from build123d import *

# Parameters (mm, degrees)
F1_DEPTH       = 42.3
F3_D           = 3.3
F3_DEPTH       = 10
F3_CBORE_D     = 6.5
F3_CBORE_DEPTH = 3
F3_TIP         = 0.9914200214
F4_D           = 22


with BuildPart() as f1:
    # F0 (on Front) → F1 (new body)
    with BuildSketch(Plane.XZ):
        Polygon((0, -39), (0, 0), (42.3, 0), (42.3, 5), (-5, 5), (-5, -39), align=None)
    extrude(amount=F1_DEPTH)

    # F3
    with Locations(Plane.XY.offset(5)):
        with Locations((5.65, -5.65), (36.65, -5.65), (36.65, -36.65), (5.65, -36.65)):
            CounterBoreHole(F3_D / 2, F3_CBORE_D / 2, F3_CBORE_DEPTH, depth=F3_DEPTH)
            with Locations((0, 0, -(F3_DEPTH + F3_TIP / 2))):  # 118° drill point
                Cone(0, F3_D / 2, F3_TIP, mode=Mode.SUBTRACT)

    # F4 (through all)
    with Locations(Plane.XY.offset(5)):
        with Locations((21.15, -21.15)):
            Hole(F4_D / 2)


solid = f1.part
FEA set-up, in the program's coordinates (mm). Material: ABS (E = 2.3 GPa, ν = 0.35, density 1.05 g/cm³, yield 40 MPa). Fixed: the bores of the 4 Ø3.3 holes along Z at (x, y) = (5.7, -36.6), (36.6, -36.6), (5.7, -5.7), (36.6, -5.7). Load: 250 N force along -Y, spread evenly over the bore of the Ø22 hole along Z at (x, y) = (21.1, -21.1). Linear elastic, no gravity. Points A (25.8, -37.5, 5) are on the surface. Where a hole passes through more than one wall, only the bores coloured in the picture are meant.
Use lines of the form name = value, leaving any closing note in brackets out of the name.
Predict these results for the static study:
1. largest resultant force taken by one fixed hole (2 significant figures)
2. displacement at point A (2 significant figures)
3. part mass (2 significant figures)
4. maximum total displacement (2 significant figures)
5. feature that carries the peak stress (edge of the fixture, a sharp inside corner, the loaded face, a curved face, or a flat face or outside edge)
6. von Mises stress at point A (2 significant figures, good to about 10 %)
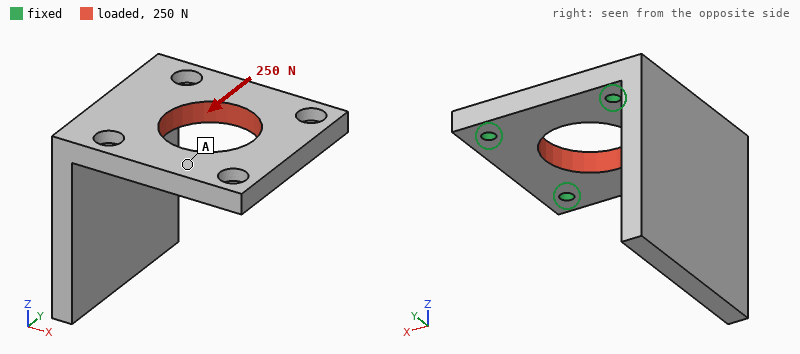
largest resultant force taken by one fixed hole = 65 N
displacement at point A = 16 µm
part mass = 17 g
maximum total displacement = 20 µm
feature that carries the peak stress = edge of the fixture
von Mises stress at point A = 0.81 MPa
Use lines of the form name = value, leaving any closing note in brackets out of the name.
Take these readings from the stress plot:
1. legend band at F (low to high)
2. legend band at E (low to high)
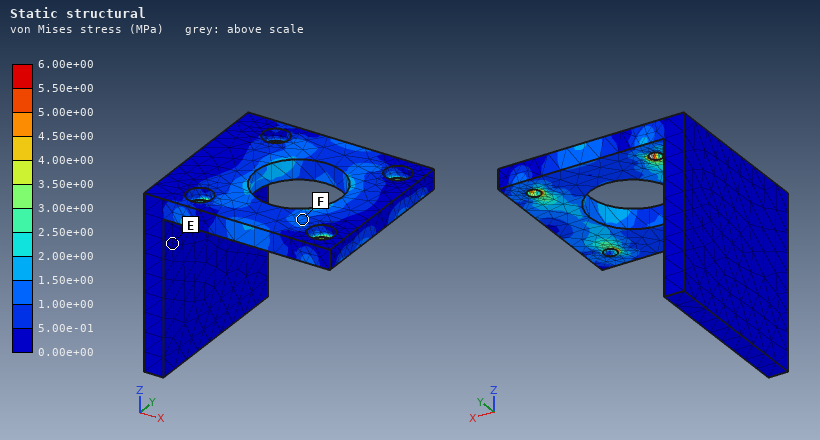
legend band at F = 1.00e+00 to 1.50e+00 MPa
legend band at E = 0.00e+00 to 5.00e-01 MPa
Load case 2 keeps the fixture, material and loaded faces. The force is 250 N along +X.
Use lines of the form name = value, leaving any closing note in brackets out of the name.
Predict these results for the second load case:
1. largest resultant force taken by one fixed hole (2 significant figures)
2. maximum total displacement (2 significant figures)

largest resultant force taken by one fixed hole = 64 N
maximum total displacement = 42 µm
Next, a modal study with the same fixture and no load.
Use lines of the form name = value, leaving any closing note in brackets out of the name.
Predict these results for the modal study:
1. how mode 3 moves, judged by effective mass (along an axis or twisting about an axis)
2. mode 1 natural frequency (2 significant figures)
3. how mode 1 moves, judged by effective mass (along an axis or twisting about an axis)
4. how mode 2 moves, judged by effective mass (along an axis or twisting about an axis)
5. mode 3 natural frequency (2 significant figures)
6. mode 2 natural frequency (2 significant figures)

how mode 3 moves, judged by effective mass = along Y
mode 1 natural frequency = 450 Hz
how mode 1 moves, judged by effective mass = along X
how mode 2 moves, judged by effective mass = along Y
mode 3 natural frequency = 1700 Hz
mode 2 natural frequency = 1300 Hz
